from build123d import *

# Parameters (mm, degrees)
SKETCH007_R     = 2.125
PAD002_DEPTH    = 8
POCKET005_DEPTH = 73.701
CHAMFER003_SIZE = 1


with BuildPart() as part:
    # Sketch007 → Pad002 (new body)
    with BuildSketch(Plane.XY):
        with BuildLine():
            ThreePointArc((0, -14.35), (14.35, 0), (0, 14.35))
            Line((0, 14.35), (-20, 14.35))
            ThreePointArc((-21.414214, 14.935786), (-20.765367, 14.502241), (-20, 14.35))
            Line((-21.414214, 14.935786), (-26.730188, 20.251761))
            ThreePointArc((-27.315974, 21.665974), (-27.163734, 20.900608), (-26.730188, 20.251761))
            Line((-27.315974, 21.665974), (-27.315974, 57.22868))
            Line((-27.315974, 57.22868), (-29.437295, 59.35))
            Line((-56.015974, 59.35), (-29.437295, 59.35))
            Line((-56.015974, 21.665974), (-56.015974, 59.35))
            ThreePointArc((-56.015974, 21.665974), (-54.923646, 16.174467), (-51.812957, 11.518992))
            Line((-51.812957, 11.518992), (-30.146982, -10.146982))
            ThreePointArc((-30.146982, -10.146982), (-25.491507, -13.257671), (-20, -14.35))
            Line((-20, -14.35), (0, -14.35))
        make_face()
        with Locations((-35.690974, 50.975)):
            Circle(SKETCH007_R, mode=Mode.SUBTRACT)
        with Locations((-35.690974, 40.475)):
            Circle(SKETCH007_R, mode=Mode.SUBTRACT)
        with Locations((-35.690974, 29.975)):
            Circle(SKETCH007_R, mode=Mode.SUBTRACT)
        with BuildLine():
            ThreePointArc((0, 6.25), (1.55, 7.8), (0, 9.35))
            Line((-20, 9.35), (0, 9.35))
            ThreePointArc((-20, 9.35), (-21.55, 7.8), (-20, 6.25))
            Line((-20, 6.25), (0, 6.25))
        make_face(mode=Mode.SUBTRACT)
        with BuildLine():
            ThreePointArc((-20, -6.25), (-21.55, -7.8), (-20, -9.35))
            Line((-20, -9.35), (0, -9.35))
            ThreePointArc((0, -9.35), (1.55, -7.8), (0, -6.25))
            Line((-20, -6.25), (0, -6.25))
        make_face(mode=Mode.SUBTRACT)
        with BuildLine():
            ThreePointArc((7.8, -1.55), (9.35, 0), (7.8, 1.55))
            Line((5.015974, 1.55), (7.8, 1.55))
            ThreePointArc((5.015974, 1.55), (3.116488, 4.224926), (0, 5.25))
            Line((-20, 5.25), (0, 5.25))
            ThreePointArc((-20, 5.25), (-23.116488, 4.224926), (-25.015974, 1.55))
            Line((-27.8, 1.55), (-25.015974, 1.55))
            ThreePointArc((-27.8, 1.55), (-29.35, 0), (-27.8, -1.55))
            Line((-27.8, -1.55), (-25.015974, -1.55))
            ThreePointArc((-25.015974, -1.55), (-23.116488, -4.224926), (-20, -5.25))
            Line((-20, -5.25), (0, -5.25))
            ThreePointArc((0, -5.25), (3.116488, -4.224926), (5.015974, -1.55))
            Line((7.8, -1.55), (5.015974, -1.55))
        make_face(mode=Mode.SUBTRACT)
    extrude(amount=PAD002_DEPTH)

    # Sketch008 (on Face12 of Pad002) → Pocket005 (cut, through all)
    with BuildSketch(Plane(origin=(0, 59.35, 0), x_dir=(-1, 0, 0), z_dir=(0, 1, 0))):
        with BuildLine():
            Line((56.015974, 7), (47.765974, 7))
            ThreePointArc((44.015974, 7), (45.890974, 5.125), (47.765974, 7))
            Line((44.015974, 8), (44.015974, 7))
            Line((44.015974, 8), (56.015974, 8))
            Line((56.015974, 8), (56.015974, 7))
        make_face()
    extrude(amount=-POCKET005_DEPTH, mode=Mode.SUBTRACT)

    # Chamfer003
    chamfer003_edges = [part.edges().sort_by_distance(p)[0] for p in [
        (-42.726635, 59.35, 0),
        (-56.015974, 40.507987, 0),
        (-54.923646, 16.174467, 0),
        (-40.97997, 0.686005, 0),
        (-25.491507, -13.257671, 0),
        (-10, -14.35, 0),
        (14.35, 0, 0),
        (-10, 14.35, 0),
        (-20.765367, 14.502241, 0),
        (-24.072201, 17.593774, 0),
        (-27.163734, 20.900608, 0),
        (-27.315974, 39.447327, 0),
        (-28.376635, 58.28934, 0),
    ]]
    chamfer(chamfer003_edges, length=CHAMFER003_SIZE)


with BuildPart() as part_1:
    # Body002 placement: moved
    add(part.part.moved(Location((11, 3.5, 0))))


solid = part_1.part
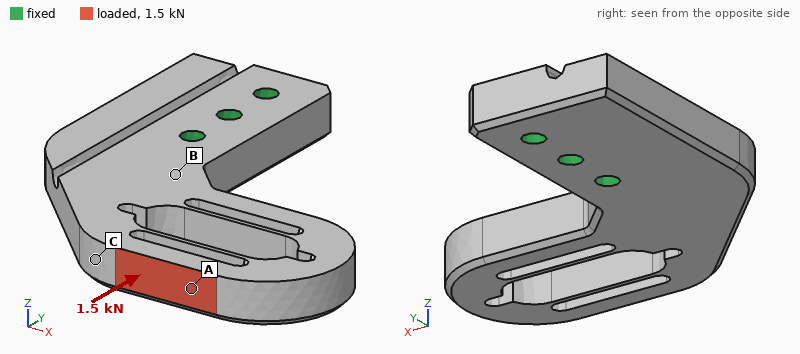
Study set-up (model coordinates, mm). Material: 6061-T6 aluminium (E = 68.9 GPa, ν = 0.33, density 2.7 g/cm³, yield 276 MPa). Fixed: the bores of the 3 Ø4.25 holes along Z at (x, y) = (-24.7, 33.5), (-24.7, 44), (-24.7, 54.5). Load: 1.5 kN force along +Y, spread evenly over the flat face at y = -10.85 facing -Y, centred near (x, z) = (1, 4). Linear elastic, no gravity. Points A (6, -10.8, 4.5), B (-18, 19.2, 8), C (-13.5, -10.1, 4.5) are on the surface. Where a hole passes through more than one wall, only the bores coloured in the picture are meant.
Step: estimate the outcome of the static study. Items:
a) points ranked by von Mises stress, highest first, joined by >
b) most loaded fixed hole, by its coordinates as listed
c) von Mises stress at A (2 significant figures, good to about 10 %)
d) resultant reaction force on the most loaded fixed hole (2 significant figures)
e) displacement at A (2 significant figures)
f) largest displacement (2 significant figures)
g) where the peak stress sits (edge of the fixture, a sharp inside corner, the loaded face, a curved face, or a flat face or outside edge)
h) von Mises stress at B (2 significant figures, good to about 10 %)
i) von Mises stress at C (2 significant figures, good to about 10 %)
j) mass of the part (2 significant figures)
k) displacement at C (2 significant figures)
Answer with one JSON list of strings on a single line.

["A > C > B", "(-24.7, 33.5)", "110 MPa", "2.5 kN", "0.32 mm", "0.37 mm", "a curved face", "29 MPa", "70 MPa", "46 g", "0.17 mm"]
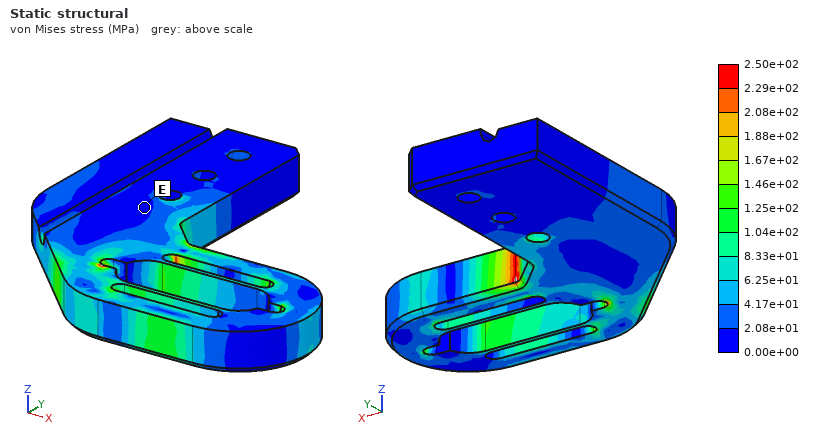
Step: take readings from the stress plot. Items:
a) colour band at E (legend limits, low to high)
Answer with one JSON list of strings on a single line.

["0.00e+00 to 2.08e+01 MPa"]
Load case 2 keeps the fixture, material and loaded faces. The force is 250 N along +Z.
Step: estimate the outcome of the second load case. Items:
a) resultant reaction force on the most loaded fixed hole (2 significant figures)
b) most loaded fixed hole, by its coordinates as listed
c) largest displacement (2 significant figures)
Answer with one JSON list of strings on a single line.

["540 N", "(-24.7, 33.5)", "0.30 mm"]
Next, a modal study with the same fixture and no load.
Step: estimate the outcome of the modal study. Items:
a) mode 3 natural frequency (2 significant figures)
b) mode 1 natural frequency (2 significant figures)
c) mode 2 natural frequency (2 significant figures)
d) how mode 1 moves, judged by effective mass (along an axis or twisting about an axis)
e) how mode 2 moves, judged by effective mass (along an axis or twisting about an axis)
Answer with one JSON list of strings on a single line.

["4000 Hz", "1600 Hz", "2900 Hz", "along Z", "along Y"]
